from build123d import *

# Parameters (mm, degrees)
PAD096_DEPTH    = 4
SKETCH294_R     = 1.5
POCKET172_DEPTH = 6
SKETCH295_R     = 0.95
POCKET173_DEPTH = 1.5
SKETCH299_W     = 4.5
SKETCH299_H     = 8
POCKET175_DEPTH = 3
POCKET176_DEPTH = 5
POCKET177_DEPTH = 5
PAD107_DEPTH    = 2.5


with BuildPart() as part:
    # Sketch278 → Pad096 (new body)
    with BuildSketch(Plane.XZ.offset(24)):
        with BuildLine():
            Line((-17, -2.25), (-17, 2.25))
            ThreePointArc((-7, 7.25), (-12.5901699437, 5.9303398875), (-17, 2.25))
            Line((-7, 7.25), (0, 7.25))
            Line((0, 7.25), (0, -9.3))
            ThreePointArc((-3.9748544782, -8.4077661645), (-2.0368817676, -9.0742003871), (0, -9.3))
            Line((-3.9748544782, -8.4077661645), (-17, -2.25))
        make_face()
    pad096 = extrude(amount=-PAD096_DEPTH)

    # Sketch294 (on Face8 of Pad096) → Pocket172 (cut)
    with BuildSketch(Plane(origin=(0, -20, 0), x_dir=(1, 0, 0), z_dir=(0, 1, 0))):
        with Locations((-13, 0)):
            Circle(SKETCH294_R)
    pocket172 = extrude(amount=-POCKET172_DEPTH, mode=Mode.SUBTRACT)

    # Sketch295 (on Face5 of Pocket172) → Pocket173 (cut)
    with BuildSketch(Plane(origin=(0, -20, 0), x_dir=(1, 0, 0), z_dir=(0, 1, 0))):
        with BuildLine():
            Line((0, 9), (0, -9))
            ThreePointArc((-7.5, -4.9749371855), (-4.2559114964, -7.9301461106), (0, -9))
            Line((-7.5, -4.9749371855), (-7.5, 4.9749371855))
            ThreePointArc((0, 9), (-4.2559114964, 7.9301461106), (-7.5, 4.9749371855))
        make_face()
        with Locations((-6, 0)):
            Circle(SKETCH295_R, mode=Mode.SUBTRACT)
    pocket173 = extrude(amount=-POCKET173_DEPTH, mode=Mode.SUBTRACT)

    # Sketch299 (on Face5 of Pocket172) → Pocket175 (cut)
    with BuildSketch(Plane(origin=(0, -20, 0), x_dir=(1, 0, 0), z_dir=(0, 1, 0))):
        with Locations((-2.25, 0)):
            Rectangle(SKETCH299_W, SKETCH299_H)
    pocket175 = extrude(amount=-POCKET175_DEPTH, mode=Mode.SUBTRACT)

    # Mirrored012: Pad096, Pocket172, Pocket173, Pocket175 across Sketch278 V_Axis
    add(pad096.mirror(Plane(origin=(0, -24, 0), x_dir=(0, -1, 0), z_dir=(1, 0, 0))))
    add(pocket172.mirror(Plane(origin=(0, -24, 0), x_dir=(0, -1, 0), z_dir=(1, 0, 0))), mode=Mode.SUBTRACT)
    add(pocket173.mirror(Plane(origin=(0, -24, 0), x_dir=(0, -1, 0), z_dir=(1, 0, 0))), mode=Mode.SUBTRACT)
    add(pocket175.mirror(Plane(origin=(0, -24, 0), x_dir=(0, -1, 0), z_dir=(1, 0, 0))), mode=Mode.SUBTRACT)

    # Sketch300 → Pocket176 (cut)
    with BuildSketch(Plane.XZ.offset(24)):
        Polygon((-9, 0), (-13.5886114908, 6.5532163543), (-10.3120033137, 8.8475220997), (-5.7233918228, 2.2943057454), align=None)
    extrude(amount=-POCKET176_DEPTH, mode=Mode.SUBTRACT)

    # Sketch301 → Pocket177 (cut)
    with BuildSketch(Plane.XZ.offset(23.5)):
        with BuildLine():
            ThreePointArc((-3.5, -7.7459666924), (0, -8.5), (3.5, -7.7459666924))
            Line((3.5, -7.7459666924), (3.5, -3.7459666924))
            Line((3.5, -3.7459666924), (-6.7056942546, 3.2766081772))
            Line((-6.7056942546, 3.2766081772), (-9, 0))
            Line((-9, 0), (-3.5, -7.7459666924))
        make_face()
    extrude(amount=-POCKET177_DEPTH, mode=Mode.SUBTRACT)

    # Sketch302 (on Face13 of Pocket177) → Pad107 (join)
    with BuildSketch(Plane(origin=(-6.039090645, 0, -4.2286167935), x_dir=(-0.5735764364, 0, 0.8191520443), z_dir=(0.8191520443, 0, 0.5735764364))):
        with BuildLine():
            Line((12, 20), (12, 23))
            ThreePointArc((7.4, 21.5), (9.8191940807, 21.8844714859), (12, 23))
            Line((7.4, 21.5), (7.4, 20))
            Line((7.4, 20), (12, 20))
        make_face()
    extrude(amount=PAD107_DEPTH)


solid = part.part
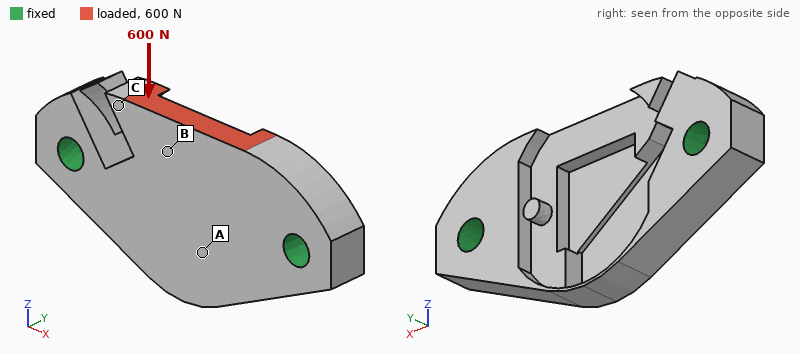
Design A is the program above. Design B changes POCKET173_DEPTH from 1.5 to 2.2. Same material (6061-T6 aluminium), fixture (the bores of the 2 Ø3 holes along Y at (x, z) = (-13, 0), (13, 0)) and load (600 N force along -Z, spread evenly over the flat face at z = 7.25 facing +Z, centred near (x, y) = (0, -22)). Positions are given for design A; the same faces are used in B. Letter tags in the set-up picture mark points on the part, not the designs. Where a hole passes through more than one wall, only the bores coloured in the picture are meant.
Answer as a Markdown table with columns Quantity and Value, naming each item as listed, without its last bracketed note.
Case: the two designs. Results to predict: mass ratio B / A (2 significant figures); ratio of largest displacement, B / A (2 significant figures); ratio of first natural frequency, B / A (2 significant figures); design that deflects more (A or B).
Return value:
| Quantity | Value |
|---|---|
| mass ratio B / A | 0.94 |
| ratio of largest displacement, B / A | 1.6 |
| ratio of first natural frequency, B / A | 0.86 |
| design that deflects more | B |
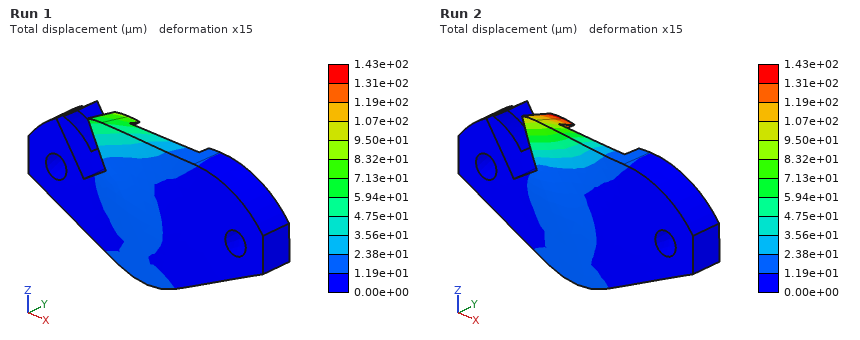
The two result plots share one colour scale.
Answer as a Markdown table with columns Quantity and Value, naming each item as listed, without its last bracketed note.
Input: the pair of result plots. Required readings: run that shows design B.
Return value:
| Quantity | Value |
|---|---|
| run that shows design B | Run 2 |
